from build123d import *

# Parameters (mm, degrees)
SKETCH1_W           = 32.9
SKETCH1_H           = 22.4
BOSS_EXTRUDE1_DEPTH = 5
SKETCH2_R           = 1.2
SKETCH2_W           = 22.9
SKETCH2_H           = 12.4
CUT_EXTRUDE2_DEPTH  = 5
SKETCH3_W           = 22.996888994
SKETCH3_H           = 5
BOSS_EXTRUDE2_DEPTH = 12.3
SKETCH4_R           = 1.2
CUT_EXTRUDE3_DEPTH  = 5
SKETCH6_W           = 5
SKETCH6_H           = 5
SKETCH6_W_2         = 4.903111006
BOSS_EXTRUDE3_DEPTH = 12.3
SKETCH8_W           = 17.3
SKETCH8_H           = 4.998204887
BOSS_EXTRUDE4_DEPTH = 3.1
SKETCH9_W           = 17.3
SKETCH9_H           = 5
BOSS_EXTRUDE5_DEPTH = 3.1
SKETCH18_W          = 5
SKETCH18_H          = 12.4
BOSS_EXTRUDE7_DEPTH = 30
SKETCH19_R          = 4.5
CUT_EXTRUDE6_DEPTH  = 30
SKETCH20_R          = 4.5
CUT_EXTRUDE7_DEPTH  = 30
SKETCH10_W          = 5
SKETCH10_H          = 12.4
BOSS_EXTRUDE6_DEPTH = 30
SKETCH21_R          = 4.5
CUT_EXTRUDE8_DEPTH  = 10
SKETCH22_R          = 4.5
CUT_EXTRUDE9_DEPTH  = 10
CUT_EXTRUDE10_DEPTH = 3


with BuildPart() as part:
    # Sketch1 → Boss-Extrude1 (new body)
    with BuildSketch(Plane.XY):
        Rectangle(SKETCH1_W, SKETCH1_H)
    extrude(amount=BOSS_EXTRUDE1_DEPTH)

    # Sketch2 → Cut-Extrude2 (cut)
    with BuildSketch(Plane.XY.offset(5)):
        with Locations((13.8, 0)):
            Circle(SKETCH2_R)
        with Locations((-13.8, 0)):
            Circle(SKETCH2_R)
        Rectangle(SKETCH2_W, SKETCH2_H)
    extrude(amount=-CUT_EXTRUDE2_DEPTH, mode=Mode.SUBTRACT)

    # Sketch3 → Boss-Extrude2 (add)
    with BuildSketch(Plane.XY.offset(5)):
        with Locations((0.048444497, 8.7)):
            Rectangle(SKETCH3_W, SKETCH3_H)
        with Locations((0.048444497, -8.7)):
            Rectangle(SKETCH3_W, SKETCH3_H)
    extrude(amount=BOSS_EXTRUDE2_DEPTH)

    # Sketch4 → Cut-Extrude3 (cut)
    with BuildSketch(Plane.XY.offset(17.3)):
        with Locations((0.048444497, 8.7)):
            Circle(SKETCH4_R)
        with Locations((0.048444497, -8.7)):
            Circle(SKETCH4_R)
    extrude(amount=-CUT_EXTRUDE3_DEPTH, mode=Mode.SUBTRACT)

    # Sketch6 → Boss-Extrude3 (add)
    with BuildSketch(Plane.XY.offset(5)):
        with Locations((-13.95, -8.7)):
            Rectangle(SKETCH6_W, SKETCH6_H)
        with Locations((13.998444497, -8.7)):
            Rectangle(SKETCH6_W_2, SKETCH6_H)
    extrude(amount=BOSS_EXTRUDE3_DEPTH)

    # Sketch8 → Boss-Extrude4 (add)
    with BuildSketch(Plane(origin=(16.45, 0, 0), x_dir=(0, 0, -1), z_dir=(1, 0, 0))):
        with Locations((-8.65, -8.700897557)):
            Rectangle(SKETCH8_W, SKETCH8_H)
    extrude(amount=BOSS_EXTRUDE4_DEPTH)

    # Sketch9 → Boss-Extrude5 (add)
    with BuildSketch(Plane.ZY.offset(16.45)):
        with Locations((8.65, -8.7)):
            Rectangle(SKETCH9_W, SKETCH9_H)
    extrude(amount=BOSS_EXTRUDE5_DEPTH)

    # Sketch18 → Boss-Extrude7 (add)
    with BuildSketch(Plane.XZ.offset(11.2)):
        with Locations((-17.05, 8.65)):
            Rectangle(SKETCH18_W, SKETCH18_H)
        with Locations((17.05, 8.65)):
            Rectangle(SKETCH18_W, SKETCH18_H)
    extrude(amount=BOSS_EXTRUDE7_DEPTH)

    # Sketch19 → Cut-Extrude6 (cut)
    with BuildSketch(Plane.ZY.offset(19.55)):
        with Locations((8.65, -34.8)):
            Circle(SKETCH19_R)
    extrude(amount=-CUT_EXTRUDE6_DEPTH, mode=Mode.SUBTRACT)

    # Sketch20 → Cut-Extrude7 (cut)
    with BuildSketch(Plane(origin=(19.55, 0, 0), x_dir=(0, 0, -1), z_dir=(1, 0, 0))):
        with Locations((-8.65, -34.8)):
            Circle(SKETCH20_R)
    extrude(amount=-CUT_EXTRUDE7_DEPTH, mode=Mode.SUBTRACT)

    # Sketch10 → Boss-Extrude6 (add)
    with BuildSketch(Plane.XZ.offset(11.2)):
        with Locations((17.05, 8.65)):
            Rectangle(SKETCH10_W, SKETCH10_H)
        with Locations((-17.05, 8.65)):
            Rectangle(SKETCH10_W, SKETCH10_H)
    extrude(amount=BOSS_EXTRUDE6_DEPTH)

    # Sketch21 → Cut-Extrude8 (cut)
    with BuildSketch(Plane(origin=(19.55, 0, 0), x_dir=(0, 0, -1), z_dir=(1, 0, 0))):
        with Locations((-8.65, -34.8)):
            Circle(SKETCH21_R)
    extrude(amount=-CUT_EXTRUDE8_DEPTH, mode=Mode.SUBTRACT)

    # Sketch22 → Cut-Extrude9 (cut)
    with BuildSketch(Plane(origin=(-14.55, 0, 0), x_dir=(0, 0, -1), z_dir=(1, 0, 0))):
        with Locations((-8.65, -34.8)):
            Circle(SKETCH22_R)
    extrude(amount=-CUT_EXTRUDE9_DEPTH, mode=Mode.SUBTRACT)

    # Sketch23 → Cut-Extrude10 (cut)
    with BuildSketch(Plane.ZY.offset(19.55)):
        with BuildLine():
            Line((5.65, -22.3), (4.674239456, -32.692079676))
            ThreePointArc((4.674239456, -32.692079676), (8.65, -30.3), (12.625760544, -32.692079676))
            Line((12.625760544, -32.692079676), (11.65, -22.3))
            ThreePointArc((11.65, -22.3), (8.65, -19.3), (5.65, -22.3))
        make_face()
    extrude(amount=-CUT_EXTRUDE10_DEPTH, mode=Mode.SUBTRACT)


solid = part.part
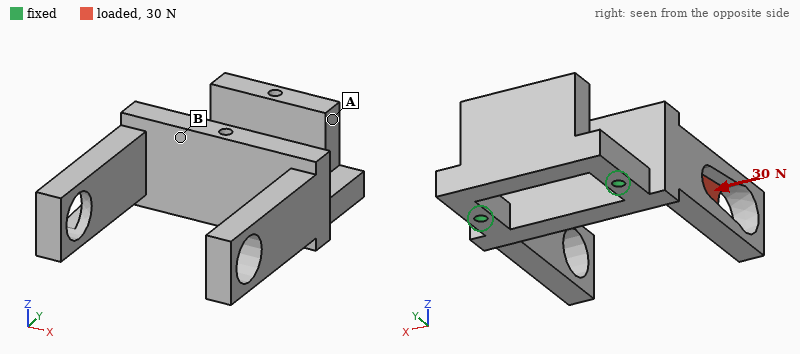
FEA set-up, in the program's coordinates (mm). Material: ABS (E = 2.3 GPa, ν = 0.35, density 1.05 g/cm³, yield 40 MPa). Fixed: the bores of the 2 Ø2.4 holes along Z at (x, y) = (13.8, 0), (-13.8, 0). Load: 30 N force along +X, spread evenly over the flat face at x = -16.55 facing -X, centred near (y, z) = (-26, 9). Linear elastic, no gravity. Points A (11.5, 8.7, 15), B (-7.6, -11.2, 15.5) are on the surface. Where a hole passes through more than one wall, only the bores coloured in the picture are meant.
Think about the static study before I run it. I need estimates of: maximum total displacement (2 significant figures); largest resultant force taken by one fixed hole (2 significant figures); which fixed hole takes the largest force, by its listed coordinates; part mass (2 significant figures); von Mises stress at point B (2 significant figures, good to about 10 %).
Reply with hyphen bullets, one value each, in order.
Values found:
- 0.72 mm
- 41 N
- (13.8, 0)
- 9.5 g
- 3.7 MPa
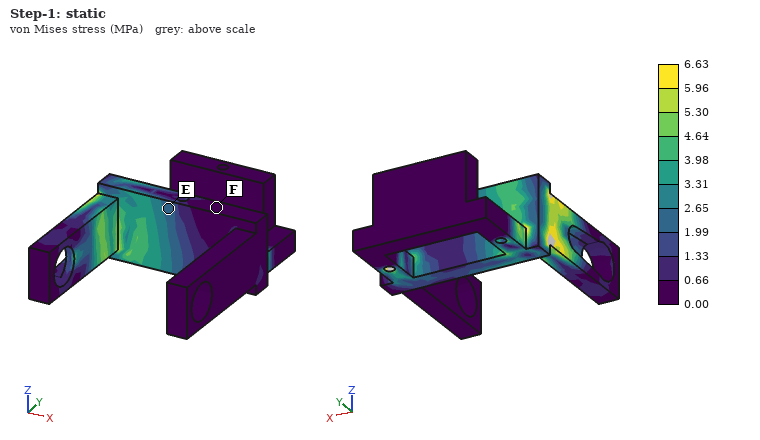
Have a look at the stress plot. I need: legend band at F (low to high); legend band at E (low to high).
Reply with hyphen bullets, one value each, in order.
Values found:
- 0.00 to 0.66 MPa
- 1.99 to 2.65 MPa
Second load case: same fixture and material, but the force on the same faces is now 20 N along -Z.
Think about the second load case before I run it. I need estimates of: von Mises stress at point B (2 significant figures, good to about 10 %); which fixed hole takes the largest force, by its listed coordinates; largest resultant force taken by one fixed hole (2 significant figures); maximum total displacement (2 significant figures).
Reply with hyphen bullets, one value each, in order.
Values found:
- 1.7 MPa
- (-13.8, 0)
- 21 N
- 0.79 mm
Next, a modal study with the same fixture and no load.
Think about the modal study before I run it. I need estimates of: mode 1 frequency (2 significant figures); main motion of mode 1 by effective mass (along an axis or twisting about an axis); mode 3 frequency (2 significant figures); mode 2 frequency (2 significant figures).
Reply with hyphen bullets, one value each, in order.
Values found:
- 630 Hz
- along Z
- 1100 Hz
- 980 Hz
